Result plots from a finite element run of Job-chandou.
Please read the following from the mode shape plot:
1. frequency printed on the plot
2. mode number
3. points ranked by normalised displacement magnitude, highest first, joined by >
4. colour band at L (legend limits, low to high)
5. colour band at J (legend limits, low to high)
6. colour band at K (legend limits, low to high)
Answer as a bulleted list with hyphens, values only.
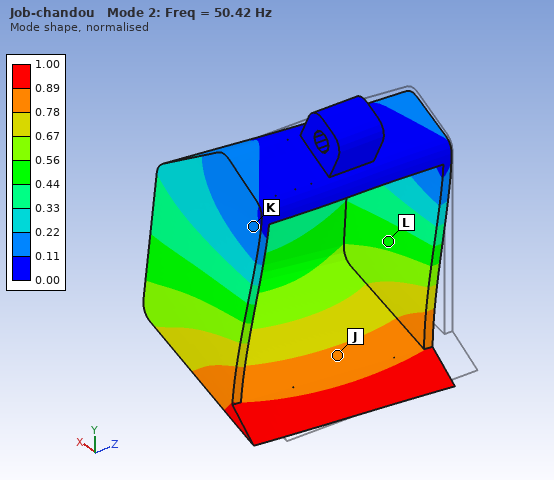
- 50.42 Hz
- 2
- J > L > K
- 0.44 to 0.56
- 0.78 to 0.89
- 0.11 to 0.22
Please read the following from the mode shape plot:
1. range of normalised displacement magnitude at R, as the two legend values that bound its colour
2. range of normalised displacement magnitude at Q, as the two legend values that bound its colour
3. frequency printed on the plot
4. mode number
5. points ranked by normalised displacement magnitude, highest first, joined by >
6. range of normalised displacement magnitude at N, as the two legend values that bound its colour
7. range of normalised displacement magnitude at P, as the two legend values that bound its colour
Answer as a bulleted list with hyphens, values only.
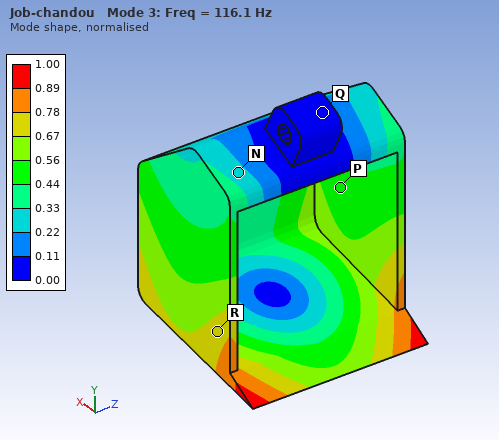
- 0.67 to 0.78
- 0.00 to 0.11
- 116.1 Hz
- 3
- R > P > N > Q
- 0.22 to 0.33
- 0.44 to 0.56
